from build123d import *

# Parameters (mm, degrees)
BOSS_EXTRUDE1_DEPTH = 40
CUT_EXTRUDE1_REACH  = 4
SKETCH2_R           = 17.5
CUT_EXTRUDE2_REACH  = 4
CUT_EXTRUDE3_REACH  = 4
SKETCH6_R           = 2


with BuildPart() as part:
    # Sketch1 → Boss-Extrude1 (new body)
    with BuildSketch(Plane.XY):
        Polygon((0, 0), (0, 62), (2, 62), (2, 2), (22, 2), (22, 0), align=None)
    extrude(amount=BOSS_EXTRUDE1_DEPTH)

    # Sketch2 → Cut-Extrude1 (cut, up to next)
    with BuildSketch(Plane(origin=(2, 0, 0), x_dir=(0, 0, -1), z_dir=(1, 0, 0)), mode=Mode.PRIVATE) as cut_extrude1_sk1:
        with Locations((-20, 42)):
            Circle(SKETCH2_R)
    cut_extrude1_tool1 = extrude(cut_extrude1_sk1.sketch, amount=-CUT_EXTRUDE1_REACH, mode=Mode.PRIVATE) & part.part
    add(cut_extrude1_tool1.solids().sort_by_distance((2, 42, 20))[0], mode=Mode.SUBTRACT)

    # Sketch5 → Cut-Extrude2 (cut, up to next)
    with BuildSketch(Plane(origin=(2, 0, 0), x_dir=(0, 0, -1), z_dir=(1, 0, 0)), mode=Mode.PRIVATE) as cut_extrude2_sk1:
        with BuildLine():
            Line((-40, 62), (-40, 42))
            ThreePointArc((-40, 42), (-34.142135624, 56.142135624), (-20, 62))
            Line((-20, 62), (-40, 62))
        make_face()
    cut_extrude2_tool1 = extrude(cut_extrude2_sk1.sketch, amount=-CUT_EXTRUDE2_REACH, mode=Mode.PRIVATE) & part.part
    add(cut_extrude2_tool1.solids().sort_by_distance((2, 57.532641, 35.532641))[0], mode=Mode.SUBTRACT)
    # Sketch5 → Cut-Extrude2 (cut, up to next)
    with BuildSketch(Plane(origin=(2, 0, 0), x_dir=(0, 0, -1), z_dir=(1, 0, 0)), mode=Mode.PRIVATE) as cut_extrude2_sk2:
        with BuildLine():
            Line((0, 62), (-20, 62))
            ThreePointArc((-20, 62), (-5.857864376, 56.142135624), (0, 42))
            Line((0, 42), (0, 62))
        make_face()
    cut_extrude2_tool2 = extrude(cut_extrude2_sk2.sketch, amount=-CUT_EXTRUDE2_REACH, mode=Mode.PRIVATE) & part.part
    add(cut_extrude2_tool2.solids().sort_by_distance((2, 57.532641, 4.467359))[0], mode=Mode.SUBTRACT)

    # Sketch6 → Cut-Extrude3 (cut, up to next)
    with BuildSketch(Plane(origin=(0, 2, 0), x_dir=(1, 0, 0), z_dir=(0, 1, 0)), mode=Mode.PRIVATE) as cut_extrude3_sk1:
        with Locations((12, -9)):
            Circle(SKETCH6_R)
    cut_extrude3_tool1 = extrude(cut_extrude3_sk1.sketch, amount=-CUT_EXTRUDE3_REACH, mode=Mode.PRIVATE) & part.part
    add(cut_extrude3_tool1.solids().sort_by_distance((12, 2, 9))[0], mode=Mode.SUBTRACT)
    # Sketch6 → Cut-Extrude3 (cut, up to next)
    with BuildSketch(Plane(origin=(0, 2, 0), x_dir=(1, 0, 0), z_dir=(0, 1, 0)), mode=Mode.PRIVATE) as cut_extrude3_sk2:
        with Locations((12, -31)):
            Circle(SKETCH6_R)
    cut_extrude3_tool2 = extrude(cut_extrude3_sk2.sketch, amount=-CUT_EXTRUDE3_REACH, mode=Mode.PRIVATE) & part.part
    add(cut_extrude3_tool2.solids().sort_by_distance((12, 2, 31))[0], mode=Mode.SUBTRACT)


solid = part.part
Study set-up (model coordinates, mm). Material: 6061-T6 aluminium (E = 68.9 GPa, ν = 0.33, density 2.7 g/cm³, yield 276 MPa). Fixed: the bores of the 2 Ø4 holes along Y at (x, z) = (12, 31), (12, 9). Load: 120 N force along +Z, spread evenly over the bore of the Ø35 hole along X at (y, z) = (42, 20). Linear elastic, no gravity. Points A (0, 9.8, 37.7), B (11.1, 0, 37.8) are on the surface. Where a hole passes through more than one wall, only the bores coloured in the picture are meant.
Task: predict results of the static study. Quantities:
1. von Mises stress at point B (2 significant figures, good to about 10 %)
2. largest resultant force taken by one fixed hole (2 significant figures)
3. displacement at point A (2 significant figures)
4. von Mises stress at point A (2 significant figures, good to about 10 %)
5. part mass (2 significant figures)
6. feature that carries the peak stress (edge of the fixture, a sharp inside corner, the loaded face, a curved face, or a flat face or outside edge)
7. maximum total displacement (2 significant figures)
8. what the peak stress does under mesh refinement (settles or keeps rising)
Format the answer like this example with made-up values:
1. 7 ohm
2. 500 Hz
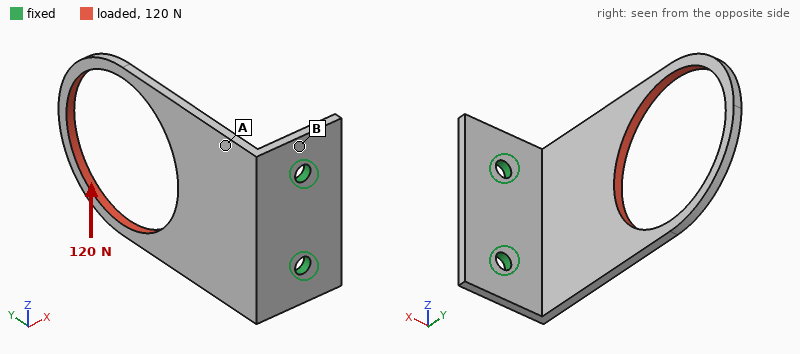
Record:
1. 58 MPa
2. 210 N
3. 0.093 mm
4. 21 MPa
5. 11 g
6. edge of the fixture
7. 0.39 mm
8. keeps rising
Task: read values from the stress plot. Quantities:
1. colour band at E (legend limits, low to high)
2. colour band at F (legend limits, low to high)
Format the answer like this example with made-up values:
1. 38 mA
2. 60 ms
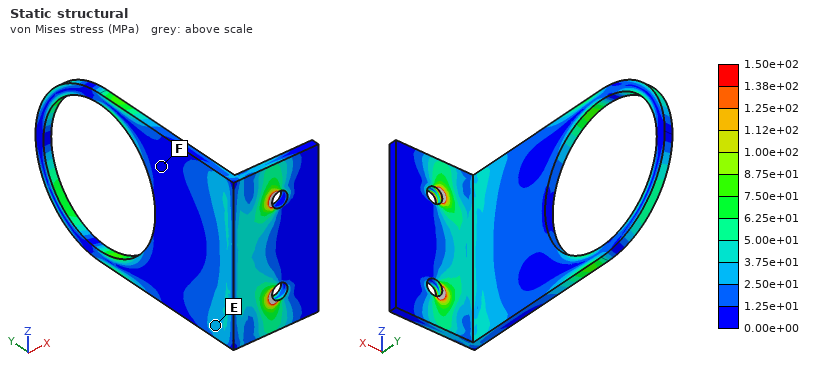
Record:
1. 2.50e+01 to 3.75e+01 MPa
2. 0.00e+00 to 1.25e+01 MPa
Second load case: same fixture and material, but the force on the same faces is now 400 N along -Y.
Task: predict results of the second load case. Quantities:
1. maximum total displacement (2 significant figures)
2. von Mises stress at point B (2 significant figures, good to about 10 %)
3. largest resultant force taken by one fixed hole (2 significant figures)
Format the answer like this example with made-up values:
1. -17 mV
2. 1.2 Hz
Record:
1. 0.73 mm
2. 64 MPa
3. 200 N
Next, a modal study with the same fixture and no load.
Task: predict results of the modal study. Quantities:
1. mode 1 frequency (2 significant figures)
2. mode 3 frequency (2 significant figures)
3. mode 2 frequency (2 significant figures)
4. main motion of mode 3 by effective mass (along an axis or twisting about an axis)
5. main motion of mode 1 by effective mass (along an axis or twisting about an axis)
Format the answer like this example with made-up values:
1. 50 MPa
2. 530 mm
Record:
1. 650 Hz
2. 1900 Hz
3. 1600 Hz
4. along X
5. along X
